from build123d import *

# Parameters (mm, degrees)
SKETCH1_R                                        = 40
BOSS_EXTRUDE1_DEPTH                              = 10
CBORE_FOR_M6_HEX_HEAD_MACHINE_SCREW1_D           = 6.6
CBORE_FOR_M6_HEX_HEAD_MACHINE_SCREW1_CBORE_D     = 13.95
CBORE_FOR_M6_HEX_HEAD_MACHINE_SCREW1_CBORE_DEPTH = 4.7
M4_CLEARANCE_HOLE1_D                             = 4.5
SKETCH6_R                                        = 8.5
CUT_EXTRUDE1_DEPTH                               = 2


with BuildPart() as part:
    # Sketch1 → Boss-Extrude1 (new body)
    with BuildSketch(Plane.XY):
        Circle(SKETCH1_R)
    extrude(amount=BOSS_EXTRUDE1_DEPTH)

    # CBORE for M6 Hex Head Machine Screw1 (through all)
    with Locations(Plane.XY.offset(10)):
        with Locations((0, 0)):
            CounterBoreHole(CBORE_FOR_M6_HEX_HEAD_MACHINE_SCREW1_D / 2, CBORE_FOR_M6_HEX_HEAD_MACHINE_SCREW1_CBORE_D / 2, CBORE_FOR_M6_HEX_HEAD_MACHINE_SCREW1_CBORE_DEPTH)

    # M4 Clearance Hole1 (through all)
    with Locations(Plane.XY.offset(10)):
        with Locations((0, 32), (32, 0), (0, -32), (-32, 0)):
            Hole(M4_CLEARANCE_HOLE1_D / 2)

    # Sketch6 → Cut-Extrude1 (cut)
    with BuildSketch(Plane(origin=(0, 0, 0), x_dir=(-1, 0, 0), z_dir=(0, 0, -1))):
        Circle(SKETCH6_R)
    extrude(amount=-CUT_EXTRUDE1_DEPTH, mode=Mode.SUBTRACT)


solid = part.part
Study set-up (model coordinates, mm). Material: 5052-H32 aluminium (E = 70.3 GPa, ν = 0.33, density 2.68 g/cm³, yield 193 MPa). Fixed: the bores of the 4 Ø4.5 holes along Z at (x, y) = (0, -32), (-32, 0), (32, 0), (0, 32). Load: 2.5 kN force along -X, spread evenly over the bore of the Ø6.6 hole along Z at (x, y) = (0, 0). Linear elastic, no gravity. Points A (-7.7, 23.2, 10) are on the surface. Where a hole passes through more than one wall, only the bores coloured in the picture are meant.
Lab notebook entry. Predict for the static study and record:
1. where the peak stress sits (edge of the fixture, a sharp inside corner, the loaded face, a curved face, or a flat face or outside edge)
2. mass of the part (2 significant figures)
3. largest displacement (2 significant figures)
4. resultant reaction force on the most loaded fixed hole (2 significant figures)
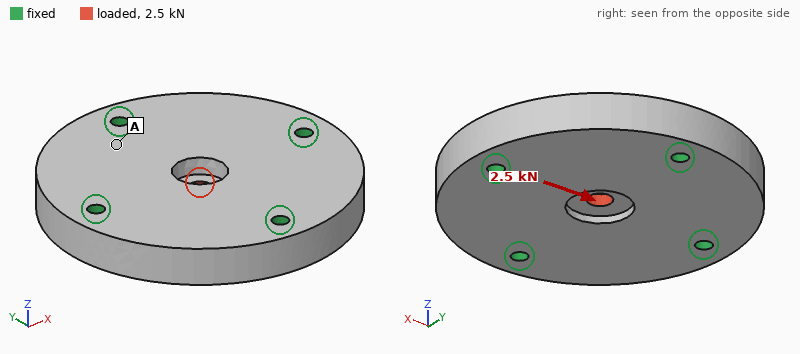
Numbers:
the loaded face
130 g
4.8 µm
820 N
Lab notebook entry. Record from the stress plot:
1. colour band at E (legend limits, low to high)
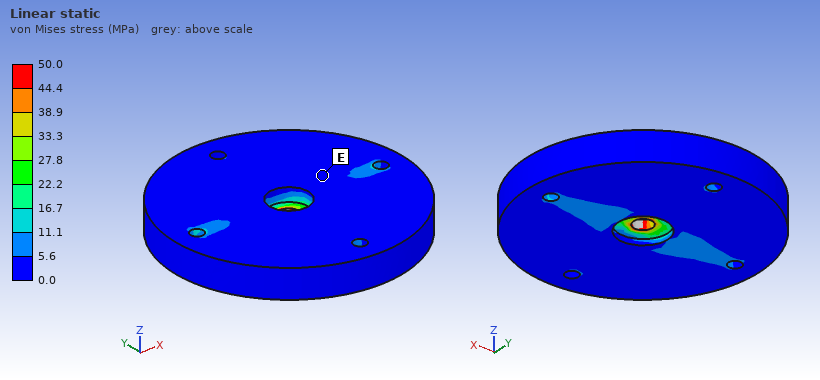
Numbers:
0.0 to 5.6 MPa
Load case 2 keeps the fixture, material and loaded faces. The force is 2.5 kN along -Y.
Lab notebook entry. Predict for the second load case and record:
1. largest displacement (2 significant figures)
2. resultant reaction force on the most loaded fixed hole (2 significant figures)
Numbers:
4.8 µm
820 N
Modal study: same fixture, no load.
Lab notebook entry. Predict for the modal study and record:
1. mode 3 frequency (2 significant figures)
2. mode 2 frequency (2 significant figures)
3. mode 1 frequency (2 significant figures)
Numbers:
16 kHz
15 kHz
14 kHz
